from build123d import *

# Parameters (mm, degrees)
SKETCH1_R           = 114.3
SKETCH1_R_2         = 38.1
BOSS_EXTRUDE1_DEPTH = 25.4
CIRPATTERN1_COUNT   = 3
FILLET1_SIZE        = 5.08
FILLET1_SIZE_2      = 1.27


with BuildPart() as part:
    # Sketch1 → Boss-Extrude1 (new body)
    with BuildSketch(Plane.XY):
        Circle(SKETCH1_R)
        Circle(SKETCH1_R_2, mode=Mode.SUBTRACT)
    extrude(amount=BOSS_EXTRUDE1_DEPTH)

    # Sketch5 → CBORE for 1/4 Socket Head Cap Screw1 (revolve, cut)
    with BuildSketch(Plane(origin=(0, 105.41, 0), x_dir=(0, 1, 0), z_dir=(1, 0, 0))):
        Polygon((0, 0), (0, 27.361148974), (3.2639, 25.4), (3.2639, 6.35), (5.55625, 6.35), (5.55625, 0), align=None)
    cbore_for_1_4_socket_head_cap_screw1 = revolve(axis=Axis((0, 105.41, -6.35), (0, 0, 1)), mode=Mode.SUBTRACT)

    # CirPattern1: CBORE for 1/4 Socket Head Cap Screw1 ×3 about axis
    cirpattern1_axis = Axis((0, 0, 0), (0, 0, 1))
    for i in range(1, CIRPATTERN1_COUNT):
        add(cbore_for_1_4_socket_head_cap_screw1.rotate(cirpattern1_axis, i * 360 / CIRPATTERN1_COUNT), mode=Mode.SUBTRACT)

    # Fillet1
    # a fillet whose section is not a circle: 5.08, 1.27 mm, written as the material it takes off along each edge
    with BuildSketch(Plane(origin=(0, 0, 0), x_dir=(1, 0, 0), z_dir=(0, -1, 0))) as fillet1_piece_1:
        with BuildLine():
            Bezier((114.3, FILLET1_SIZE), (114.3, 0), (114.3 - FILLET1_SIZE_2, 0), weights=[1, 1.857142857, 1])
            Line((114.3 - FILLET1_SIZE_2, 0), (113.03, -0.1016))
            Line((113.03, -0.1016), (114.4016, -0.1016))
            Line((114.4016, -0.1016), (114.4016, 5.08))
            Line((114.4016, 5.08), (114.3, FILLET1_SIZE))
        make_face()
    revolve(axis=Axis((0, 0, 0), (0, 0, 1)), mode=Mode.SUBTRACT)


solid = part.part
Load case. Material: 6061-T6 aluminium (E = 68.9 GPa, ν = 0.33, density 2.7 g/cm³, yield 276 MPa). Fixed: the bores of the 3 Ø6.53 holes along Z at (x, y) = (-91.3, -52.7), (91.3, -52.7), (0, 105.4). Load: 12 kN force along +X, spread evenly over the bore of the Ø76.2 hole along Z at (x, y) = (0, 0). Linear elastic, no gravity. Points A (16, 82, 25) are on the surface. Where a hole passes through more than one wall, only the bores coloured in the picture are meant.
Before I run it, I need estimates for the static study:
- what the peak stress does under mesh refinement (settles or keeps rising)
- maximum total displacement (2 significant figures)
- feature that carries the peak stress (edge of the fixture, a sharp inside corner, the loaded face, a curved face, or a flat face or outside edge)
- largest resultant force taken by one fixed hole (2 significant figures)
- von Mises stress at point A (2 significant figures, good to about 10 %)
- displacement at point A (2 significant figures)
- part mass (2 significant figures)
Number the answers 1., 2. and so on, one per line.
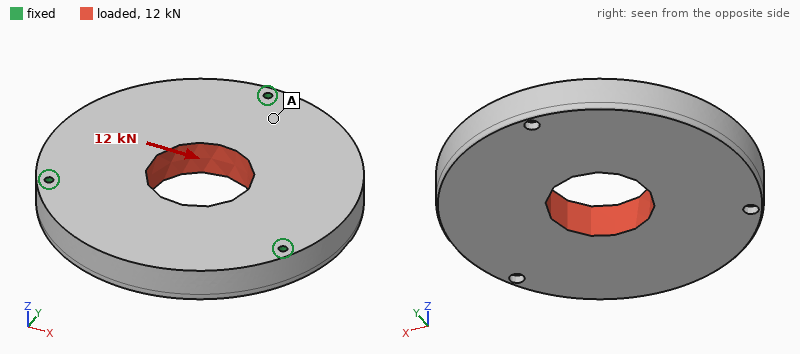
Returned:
1. keeps rising
2. 7.3 µm
3. edge of the fixture
4. 4.2 kN
5. 2.3 MPa
6. 3.2 µm
7. 2.5 kg
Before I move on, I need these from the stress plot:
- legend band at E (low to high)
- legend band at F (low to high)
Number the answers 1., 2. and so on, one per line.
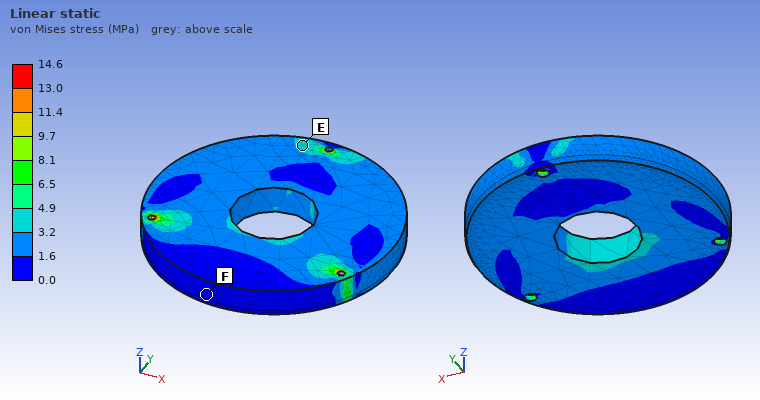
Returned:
1. 3.2 to 4.9 MPa
2. 0.0 to 1.6 MPa
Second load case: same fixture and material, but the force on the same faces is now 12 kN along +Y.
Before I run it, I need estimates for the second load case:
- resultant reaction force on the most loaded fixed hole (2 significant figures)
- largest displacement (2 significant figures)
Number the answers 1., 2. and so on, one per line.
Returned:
1. 4.1 kN
2. 7.9 µm
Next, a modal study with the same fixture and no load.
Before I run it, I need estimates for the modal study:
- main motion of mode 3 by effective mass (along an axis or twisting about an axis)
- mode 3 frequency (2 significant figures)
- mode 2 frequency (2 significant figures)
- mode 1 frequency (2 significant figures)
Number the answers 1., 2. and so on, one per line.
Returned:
1. along Z
2. 2300 Hz
3. 2000 Hz
4. 2000 Hz
